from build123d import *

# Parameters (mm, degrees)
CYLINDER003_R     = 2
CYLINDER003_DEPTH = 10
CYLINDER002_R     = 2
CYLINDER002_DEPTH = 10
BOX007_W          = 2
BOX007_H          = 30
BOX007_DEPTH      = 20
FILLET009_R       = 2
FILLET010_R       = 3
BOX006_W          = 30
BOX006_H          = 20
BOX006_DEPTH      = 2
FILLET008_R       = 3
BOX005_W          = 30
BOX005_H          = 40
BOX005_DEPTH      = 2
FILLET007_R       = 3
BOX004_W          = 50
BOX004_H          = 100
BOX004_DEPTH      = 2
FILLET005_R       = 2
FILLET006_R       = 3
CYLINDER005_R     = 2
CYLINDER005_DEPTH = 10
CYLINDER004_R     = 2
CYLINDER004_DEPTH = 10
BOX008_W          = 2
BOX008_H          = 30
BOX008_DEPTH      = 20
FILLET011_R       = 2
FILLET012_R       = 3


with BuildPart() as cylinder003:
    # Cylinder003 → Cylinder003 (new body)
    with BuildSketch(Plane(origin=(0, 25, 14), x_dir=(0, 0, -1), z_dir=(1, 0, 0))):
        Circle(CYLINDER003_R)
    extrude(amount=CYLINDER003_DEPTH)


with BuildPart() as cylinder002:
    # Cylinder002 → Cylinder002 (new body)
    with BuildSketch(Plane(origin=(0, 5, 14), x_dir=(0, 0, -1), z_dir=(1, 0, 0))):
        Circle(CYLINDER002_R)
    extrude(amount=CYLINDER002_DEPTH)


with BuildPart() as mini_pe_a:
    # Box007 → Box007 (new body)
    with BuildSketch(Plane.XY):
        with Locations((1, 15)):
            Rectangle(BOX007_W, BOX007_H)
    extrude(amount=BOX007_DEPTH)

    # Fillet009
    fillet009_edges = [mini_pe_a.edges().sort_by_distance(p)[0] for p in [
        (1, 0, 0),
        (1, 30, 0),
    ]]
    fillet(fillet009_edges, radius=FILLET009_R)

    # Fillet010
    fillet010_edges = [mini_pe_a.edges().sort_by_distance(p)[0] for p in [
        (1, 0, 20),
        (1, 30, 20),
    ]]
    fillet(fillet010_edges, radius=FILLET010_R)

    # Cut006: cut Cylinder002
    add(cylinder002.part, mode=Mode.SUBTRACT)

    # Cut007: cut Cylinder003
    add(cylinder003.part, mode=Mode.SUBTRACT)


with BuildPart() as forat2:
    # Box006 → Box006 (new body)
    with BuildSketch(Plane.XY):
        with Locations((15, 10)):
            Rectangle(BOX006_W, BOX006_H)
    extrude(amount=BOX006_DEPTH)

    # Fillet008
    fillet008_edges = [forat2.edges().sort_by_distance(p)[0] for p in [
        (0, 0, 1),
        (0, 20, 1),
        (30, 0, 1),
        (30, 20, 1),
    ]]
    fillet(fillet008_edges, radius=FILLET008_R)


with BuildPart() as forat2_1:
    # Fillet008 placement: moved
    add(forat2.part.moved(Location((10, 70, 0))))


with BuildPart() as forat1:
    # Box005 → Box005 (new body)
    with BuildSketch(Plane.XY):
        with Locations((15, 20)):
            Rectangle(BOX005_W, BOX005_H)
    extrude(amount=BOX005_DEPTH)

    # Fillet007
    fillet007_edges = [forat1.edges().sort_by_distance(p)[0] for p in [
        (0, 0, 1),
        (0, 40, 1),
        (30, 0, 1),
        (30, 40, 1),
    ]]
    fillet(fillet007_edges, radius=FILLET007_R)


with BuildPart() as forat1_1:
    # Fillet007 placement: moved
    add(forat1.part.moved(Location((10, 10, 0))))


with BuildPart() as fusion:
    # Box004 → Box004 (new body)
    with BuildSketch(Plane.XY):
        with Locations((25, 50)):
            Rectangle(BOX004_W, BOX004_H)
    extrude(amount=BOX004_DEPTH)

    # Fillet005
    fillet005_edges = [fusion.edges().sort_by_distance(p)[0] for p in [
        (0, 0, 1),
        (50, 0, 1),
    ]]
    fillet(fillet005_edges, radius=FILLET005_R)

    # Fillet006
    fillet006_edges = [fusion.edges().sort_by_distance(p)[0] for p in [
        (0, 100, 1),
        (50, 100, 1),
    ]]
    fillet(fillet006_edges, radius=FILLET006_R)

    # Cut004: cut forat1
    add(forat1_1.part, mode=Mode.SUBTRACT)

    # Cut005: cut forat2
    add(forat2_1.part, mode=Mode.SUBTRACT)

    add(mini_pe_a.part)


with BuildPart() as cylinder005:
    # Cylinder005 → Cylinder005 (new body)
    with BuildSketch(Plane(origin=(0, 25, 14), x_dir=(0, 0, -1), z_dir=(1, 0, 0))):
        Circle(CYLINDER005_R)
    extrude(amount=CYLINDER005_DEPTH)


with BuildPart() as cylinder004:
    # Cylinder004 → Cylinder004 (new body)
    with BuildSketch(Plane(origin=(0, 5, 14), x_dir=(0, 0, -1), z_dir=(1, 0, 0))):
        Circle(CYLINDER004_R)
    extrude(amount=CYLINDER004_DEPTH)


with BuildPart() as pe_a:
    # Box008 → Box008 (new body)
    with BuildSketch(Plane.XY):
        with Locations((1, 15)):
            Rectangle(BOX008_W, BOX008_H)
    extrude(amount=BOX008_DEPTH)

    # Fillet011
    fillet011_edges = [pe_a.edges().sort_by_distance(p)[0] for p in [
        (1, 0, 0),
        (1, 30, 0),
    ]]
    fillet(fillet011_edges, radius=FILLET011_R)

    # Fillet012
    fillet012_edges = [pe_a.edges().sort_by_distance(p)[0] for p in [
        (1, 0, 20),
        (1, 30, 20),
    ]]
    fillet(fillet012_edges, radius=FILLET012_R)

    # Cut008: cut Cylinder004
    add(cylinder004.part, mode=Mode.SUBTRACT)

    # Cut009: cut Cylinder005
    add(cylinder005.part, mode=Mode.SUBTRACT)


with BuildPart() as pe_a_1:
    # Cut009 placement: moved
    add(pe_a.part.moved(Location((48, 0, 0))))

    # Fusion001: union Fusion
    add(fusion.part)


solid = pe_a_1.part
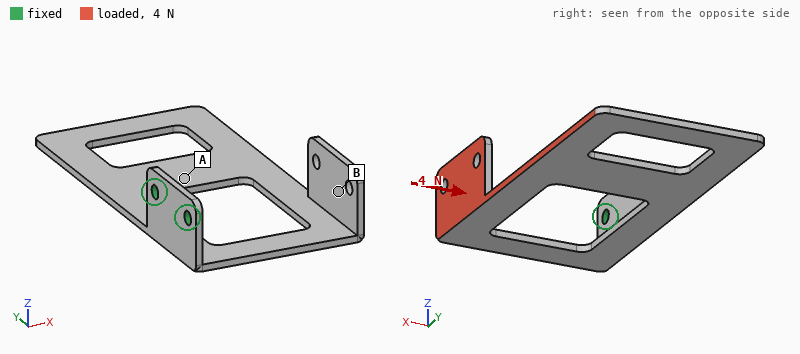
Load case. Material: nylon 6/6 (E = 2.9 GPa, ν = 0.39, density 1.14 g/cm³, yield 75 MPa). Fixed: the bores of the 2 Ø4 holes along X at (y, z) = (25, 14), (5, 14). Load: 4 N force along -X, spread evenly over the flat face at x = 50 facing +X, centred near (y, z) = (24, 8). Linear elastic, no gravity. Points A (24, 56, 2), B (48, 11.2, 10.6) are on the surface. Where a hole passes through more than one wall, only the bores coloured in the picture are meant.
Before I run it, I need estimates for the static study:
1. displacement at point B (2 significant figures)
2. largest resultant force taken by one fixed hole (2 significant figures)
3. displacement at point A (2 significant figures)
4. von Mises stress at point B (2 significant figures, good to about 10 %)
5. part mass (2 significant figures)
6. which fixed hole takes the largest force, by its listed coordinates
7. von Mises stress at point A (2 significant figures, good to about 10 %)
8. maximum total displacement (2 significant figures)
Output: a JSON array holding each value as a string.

["0.93 mm", "3.7 N", "0.30 mm", "0.35 MPa", "9.7 g", "(25, 14)", "0.91 MPa", "1.2 mm"]
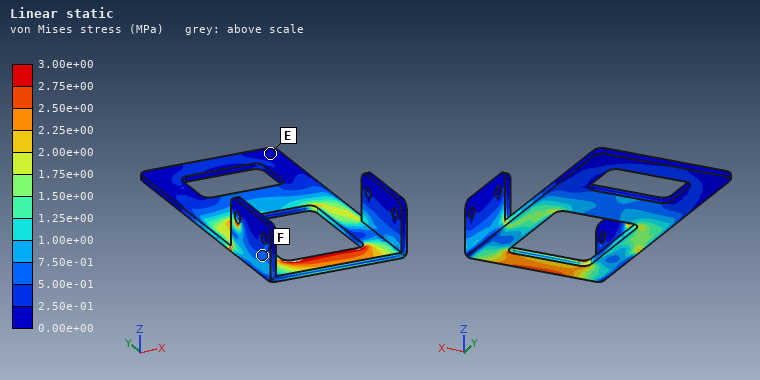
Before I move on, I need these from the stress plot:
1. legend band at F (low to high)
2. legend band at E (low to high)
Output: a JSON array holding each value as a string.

["5.00e-01 to 7.50e-01 MPa", "0.00e+00 to 2.50e-01 MPa"]
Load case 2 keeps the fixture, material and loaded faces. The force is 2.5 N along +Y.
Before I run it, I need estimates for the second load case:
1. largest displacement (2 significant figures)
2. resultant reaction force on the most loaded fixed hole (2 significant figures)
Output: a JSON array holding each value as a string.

["1.2 mm", "5.9 N"]
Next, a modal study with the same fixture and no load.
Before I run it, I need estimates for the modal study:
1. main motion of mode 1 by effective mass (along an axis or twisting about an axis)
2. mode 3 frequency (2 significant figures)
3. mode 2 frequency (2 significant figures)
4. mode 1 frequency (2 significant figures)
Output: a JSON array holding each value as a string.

["along Z", "140 Hz", "92 Hz", "50 Hz"]
